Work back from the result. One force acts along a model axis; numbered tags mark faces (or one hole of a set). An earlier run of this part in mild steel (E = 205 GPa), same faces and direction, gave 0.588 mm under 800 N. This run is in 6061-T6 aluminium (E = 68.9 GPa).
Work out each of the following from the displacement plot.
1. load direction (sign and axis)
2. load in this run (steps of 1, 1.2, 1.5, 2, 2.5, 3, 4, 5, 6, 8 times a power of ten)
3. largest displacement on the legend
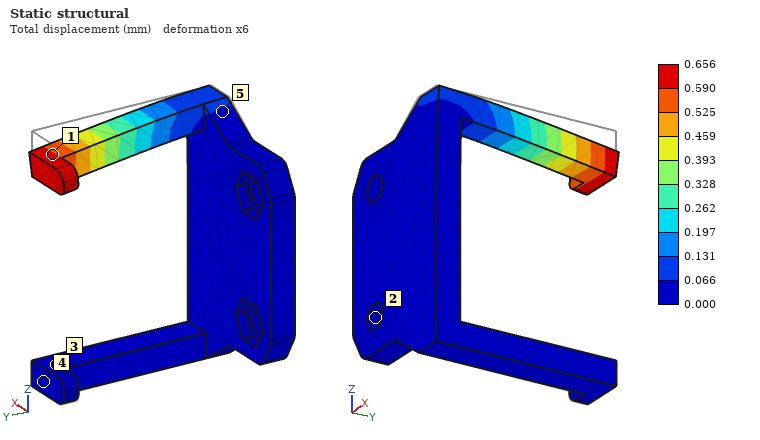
-Z
300 N
0.656 mm
